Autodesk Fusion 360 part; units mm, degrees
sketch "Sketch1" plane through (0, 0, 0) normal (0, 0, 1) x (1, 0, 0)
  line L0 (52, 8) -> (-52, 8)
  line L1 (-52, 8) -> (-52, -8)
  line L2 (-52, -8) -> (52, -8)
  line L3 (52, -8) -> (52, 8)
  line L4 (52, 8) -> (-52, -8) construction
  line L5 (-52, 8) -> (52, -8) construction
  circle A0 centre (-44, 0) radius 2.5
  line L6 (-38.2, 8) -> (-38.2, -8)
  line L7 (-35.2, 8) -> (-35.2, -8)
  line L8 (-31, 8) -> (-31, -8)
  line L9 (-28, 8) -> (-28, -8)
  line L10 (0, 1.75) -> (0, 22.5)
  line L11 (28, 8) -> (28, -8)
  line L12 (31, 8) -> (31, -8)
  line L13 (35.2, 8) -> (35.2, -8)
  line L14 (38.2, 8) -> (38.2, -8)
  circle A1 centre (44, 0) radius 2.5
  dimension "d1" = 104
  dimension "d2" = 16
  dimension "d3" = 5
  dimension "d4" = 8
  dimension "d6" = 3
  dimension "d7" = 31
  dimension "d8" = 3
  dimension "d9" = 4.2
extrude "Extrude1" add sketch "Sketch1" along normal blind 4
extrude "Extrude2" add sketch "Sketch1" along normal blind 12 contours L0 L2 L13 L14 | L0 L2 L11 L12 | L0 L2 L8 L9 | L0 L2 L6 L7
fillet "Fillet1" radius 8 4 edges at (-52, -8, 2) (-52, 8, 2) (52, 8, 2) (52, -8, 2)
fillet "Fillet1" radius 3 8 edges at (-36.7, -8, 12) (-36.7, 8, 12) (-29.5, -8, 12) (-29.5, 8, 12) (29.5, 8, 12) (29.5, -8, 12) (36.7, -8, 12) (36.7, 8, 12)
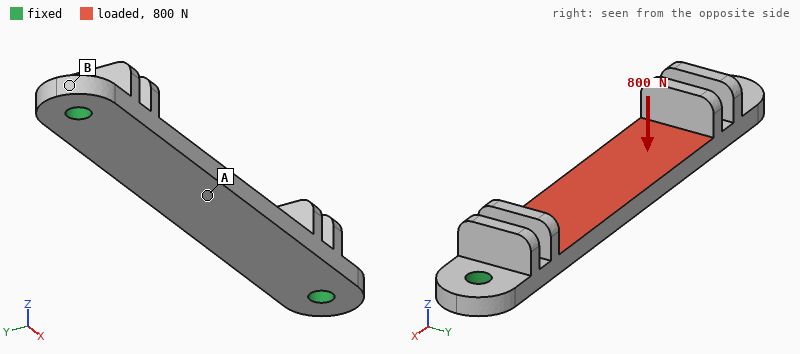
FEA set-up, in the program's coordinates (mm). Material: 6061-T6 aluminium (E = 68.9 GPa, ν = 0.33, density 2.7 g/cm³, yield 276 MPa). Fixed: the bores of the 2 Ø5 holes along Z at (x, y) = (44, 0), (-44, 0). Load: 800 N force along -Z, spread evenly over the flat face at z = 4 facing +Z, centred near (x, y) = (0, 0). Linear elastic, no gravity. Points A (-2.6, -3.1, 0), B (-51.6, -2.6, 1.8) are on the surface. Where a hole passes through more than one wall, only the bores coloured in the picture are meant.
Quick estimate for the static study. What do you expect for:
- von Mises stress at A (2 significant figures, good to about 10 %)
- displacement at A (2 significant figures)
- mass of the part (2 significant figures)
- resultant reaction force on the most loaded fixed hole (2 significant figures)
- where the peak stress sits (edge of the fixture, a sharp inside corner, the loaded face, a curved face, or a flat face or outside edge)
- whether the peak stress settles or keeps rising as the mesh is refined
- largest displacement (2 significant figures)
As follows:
93 MPa
0.31 mm
21 g
400 N
edge of the fixture
keeps rising
0.31 mm
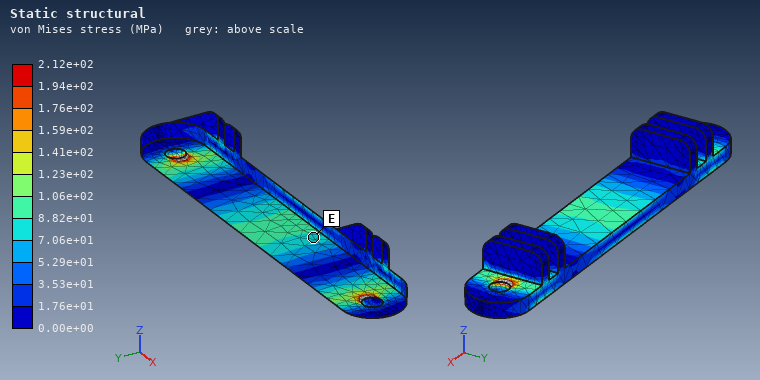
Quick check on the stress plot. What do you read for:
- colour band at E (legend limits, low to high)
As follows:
7.06e+01 to 8.82e+01 MPa
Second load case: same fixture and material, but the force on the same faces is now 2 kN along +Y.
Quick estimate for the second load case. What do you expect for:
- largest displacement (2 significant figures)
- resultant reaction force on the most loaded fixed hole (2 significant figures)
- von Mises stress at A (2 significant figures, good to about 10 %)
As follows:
0.12 mm
1.0 kN
35 MPa
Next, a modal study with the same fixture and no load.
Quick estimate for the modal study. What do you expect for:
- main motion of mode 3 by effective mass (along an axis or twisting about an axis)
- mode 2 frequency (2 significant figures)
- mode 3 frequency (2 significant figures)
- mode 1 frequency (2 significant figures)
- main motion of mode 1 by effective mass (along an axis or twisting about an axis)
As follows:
along Y
7000 Hz
7200 Hz
2800 Hz
along Z
